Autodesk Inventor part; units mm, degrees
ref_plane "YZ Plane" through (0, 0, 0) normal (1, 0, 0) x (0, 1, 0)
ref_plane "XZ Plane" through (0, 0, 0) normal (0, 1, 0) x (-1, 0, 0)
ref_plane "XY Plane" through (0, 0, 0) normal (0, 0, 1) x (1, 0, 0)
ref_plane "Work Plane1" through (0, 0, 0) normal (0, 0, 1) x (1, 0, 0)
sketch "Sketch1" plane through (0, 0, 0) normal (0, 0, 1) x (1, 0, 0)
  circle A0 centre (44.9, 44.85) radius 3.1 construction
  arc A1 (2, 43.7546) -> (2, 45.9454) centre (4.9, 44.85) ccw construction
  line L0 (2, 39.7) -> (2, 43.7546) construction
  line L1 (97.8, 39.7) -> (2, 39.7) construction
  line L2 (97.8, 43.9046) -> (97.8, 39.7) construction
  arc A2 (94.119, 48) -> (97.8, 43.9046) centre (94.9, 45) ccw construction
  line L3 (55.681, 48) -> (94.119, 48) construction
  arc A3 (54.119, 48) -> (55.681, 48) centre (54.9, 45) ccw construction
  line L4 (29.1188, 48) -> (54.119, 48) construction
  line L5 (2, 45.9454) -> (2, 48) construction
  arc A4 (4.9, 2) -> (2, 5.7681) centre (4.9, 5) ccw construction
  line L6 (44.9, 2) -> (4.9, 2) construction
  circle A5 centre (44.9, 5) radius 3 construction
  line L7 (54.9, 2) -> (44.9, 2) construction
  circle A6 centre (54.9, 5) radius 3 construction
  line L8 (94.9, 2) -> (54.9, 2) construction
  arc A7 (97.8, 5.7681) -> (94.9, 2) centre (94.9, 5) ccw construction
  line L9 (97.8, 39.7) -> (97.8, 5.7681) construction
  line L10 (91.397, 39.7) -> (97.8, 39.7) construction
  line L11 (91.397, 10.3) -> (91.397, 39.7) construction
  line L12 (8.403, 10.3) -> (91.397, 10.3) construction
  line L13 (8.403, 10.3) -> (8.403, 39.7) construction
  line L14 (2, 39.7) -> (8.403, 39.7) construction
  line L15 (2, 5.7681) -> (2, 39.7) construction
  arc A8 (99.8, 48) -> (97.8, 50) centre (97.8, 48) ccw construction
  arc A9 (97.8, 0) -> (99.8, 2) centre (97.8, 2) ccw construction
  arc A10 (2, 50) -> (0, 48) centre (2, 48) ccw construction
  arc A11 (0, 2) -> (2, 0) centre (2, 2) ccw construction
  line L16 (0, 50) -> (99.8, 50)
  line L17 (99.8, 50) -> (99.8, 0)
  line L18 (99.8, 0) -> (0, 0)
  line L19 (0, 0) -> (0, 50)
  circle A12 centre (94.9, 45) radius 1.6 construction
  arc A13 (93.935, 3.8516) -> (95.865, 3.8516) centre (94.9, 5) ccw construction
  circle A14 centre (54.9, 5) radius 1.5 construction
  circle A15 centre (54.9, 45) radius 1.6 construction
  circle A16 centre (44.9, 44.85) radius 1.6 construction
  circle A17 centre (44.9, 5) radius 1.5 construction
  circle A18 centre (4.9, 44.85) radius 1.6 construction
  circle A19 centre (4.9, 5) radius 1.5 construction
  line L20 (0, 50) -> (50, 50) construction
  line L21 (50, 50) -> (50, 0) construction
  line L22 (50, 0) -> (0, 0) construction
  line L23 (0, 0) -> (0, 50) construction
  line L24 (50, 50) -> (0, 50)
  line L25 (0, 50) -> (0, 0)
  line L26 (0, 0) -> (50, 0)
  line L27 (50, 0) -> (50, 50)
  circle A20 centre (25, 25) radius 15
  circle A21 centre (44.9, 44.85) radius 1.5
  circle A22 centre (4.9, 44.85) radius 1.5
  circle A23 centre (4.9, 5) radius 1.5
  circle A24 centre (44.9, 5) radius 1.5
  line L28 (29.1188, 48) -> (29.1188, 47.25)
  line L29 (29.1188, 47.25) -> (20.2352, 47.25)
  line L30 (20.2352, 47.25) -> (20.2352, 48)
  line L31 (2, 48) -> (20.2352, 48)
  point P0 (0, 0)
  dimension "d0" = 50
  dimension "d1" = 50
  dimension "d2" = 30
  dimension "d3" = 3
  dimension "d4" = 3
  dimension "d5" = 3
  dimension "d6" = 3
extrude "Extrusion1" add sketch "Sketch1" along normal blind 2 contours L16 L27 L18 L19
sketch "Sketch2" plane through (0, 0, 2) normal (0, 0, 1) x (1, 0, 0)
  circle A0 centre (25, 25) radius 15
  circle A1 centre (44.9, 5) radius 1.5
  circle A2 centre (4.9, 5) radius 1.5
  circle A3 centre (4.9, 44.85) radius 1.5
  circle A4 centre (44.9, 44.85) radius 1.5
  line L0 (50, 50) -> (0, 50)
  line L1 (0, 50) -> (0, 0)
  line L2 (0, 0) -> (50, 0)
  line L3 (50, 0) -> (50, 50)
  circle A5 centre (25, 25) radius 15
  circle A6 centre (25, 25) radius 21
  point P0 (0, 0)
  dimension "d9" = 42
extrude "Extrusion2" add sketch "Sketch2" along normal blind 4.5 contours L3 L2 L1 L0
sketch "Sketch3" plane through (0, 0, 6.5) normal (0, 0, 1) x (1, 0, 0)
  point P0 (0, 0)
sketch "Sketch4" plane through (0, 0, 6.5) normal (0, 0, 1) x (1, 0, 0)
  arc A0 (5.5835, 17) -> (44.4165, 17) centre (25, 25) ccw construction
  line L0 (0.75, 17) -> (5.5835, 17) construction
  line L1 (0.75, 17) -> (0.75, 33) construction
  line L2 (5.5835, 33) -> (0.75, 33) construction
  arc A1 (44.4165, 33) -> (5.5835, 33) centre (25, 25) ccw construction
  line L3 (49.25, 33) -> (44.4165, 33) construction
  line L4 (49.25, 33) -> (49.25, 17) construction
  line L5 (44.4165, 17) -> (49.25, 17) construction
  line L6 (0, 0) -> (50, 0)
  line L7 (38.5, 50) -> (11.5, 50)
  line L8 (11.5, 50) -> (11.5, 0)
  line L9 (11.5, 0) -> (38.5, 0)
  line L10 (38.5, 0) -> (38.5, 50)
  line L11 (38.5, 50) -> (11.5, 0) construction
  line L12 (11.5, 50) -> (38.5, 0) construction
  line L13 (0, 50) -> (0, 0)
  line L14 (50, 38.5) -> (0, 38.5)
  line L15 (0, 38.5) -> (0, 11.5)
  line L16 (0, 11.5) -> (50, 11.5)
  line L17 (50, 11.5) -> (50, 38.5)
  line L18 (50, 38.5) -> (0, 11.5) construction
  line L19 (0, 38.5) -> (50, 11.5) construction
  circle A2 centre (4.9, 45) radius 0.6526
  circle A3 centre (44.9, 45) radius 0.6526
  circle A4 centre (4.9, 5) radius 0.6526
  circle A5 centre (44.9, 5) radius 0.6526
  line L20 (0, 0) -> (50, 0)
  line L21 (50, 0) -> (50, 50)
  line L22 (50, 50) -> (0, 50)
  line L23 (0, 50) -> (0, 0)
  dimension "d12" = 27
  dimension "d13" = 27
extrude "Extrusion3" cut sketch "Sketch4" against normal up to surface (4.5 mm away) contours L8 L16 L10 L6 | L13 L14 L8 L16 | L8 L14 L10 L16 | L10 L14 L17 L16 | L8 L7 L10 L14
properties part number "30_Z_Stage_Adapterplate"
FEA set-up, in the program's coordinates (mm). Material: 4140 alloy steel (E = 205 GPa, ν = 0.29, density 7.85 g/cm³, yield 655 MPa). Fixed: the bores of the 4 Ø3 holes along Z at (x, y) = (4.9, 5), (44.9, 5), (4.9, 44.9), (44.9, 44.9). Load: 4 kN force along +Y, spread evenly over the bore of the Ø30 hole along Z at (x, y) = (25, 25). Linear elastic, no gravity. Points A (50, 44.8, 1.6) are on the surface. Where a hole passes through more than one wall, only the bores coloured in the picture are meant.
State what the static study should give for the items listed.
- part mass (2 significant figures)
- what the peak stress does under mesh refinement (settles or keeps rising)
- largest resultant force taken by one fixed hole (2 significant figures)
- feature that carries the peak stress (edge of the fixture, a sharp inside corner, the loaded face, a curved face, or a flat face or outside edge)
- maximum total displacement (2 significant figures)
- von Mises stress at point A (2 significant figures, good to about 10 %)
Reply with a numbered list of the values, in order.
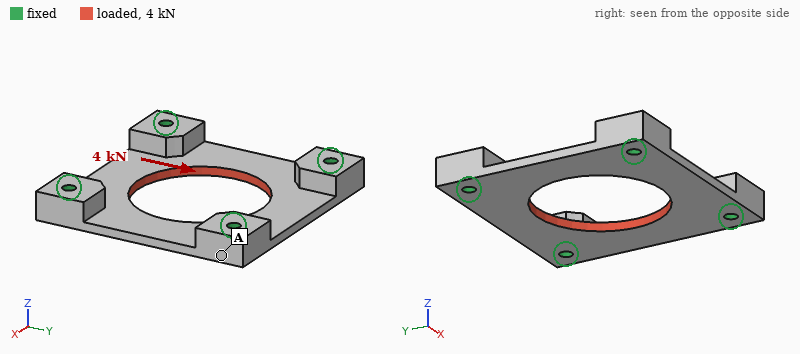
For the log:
1. 45 g
2. keeps rising
3. 1.0 kN
4. edge of the fixture
5. 7.4 µm
6. 13 MPa
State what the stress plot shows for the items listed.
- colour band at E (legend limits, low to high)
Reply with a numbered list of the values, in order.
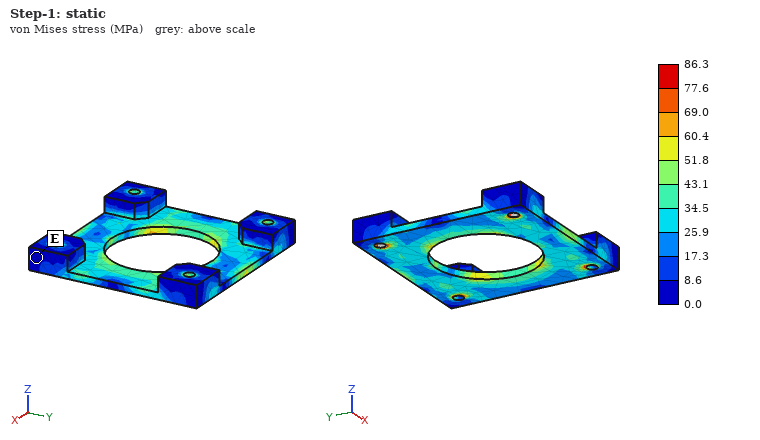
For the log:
1. 0.0 to 8.6 MPa
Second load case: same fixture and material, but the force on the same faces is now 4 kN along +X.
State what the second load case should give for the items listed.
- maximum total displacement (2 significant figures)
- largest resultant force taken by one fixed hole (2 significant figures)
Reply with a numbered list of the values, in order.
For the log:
1. 7.3 µm
2. 1.0 kN
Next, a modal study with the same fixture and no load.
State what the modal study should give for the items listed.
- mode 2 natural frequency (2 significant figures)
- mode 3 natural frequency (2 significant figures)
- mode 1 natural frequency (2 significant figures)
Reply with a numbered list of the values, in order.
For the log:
1. 12 kHz
2. 12 kHz
3. 12 kHz
